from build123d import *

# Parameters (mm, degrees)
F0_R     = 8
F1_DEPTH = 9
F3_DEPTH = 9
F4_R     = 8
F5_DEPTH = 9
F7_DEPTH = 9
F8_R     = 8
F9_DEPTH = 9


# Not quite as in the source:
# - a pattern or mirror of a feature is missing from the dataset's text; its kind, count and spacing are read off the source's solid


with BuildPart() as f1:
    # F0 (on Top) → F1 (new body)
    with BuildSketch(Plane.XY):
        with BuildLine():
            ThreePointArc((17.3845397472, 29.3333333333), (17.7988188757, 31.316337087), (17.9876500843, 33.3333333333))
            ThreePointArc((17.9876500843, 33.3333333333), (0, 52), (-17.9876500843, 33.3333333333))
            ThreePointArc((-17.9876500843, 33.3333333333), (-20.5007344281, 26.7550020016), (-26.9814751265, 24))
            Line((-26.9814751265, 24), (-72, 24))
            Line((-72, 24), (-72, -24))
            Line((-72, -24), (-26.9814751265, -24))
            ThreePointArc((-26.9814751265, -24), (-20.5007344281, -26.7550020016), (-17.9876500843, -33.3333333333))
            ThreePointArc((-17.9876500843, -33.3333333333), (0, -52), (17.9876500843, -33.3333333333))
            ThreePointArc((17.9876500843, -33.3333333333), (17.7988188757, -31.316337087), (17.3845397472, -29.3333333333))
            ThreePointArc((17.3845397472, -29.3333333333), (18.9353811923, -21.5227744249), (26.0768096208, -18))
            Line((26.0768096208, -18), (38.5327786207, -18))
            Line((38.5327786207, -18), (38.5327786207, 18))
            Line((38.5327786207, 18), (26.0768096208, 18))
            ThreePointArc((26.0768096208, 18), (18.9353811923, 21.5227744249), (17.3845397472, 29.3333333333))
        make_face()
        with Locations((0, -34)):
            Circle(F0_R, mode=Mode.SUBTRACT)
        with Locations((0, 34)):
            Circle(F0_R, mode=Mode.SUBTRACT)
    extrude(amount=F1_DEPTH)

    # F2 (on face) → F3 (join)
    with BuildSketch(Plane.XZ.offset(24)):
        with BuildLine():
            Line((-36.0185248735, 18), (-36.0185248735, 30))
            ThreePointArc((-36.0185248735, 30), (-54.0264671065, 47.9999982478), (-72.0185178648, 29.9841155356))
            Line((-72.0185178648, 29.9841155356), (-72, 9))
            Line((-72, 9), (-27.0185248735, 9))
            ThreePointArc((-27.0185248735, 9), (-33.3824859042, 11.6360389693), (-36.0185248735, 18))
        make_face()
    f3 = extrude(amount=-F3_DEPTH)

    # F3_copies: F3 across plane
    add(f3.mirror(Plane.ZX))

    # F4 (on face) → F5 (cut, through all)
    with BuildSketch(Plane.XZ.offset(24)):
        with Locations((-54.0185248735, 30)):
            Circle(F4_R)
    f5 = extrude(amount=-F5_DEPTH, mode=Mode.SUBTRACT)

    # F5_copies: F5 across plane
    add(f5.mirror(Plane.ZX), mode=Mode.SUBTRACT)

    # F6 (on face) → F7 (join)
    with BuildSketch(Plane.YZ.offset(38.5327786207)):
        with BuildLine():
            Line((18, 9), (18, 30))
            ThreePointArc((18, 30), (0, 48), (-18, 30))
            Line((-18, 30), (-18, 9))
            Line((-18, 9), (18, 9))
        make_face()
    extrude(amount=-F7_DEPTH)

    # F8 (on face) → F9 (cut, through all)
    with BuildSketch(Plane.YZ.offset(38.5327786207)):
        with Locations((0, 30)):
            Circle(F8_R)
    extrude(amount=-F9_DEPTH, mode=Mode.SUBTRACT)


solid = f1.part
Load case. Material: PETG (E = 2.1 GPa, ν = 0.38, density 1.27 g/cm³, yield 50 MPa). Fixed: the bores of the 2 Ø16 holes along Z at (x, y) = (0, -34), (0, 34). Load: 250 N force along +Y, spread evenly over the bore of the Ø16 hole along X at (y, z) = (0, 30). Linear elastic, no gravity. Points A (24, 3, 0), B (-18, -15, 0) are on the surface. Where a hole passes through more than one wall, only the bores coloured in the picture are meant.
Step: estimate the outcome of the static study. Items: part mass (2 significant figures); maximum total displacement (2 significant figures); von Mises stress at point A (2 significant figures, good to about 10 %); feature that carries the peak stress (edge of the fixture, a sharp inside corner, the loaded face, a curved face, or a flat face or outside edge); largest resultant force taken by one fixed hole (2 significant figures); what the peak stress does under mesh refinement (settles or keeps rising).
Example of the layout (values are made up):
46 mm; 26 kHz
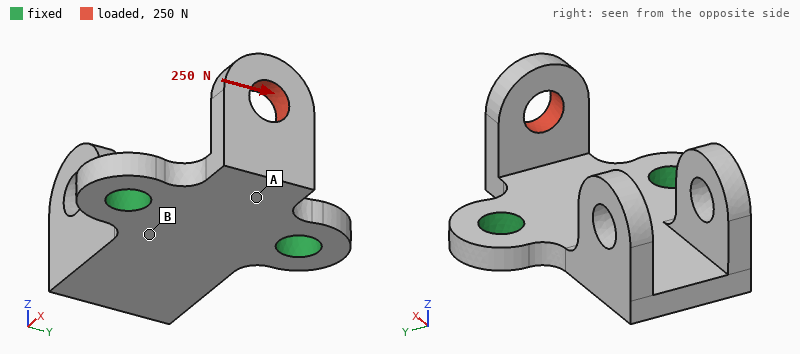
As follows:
110 g; 0.78 mm; 5.6 MPa; a sharp inside corner; 230 N; keeps rising
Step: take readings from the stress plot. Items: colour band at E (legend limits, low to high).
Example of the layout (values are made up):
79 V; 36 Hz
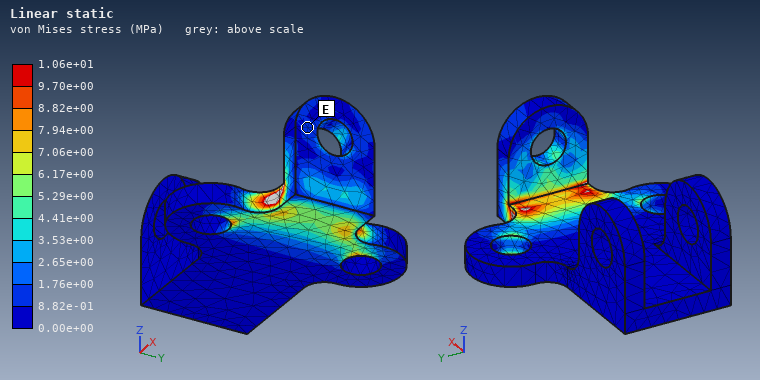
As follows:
8.82e-01 to 1.76e+00 MPa
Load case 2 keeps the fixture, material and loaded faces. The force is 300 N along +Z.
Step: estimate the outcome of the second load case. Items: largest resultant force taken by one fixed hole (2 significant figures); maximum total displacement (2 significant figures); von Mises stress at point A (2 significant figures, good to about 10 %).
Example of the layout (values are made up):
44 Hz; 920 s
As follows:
150 N; 1.5 mm; 5.9 MPa
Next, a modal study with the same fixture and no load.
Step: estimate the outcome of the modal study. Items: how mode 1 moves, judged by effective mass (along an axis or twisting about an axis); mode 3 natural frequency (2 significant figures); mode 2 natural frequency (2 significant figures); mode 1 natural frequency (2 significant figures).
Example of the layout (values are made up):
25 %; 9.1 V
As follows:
along Z; 550 Hz; 510 Hz; 250 Hz
